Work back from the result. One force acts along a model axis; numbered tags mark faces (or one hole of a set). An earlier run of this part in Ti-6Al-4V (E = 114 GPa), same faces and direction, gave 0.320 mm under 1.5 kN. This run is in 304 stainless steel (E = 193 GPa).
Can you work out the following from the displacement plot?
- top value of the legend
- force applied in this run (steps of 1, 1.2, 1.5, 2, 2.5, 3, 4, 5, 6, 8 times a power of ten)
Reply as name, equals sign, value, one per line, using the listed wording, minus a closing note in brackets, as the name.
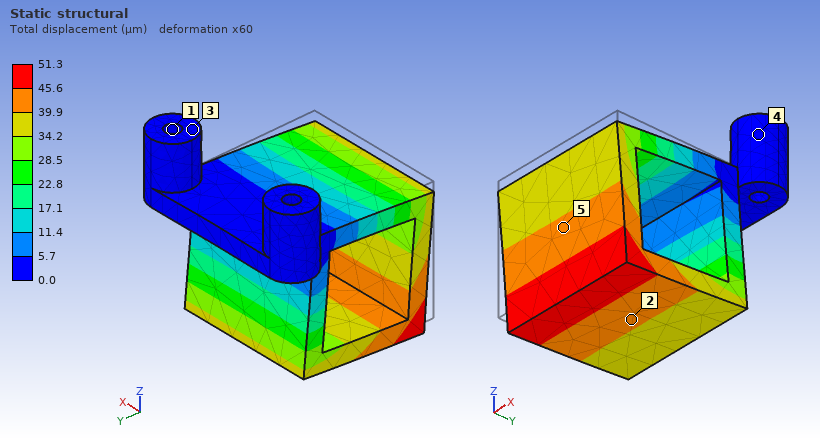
top value of the legend = 51.3 µm
force applied in this run = 400 N
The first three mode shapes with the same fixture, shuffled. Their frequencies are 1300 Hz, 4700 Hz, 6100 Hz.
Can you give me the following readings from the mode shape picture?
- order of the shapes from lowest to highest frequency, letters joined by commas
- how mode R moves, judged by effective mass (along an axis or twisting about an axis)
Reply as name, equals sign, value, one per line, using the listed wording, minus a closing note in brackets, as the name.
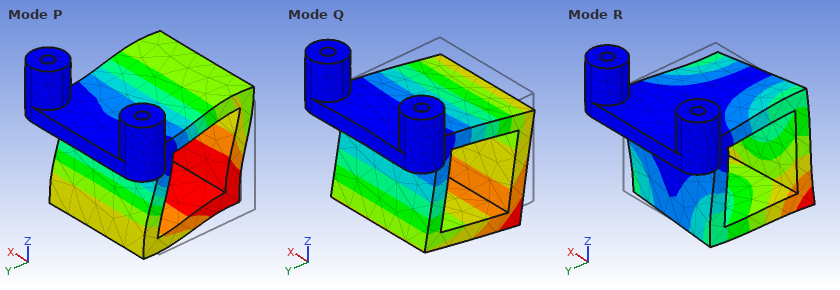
order of the shapes from lowest to highest frequency, letters joined by commas = Q, R, P
how mode R moves, judged by effective mass = along X
